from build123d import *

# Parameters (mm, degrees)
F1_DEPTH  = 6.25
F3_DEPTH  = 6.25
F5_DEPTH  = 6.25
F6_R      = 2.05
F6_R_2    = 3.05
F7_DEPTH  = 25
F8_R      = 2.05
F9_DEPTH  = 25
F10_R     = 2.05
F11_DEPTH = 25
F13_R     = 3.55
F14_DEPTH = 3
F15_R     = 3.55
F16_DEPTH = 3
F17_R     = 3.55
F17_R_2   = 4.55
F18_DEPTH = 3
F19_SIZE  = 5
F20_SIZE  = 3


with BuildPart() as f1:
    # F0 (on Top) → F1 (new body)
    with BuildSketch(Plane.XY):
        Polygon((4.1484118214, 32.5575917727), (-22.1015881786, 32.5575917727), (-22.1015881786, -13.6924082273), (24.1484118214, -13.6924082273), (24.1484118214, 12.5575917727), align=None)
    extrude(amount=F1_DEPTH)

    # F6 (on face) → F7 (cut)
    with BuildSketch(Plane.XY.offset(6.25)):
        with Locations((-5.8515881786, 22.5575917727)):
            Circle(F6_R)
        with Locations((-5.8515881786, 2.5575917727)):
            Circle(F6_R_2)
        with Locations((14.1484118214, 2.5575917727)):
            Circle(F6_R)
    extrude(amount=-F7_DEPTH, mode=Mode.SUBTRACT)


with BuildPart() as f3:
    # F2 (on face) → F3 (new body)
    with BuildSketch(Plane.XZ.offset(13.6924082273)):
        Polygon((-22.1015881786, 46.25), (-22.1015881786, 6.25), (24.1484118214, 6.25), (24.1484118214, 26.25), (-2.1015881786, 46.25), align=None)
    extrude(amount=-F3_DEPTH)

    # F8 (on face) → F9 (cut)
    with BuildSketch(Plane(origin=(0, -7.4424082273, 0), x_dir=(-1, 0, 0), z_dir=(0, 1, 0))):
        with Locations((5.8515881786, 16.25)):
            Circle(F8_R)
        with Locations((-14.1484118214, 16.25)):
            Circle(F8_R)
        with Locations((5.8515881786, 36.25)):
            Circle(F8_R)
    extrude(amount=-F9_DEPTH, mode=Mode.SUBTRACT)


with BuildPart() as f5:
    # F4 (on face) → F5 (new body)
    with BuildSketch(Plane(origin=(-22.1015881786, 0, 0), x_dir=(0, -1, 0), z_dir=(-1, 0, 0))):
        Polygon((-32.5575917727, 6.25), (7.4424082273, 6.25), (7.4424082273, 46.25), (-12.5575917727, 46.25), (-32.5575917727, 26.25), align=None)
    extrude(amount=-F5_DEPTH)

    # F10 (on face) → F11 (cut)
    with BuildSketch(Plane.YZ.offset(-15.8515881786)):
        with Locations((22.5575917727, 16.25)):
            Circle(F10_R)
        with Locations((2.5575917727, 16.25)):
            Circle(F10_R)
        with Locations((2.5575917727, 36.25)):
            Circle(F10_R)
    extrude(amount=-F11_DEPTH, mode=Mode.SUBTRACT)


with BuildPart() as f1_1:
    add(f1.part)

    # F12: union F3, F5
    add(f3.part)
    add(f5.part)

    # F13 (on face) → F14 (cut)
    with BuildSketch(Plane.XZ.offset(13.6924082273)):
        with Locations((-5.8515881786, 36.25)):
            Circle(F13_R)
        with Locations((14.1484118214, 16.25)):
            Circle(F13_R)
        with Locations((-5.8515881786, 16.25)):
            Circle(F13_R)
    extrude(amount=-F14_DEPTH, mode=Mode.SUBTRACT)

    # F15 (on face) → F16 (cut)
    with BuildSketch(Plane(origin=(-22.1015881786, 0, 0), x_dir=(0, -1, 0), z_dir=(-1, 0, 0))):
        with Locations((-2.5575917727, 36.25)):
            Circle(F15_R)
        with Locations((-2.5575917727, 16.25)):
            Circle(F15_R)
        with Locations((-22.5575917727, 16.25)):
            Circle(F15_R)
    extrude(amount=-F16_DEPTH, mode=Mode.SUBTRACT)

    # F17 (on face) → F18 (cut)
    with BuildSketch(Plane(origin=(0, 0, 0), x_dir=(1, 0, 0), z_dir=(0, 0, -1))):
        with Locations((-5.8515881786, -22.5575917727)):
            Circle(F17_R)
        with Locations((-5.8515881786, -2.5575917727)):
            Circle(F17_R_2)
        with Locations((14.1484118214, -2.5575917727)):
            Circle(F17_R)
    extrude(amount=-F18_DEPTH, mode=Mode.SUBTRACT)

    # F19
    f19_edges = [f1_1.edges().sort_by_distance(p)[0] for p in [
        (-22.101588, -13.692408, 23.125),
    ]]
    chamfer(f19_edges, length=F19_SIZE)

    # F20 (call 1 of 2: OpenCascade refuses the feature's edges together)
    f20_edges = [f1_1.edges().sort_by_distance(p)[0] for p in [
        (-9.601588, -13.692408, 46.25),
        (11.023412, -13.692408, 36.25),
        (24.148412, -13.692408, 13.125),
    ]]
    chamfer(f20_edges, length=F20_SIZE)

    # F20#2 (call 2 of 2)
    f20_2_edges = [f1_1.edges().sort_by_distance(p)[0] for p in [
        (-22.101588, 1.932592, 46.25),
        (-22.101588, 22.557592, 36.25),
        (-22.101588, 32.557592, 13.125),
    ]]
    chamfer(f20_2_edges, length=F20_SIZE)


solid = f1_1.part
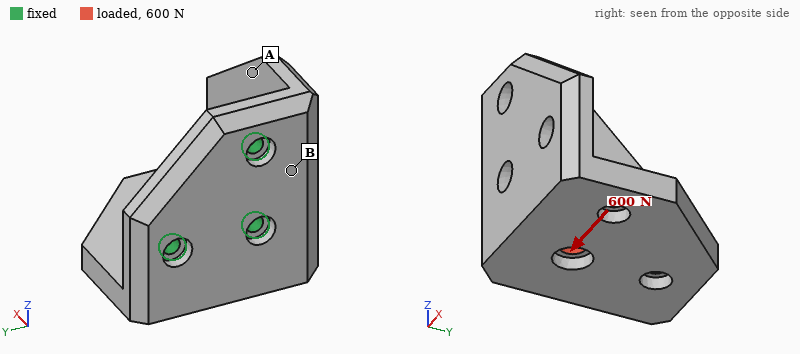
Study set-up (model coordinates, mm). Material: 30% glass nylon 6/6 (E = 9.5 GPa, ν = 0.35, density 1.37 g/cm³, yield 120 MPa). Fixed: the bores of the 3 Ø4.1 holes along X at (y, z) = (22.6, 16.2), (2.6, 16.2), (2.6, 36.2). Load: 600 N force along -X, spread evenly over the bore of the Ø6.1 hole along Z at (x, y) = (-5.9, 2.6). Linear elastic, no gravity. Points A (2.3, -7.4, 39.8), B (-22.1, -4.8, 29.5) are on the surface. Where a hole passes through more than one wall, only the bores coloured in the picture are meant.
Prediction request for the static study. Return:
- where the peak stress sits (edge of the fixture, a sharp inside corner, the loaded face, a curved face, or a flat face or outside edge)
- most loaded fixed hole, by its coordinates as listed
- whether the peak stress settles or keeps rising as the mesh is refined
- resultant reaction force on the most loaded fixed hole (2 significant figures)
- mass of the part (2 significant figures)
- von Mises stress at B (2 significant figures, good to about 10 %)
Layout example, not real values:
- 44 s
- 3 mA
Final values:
- edge of the fixture
- (2.6, 16.2)
- keeps rising
- 760 N
- 38 g
- 8.4 MPa
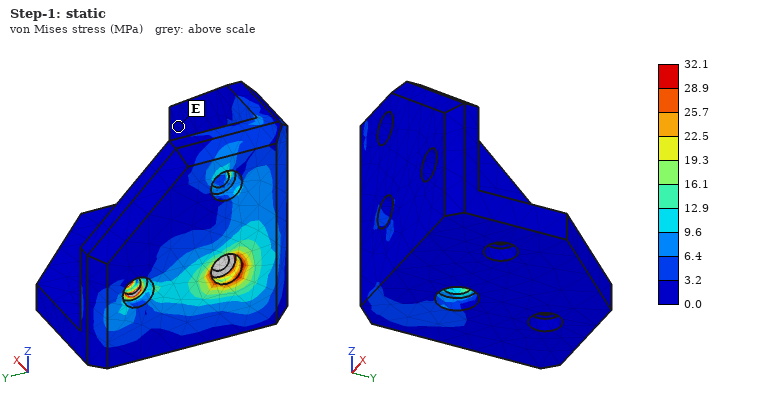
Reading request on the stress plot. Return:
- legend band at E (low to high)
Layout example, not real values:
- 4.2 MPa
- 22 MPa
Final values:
- 0.0 to 3.2 MPa
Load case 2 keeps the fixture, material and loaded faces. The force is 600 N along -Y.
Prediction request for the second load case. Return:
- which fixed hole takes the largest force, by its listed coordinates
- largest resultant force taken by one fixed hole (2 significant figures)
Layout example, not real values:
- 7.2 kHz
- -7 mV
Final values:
- (2.6, 16.2)
- 560 N
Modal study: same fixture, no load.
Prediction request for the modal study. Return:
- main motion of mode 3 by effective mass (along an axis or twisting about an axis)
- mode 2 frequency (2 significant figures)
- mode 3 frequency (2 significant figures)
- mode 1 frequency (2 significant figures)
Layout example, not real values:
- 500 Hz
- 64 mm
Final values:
- along X
- 1700 Hz
- 3600 Hz
- 1500 Hz
